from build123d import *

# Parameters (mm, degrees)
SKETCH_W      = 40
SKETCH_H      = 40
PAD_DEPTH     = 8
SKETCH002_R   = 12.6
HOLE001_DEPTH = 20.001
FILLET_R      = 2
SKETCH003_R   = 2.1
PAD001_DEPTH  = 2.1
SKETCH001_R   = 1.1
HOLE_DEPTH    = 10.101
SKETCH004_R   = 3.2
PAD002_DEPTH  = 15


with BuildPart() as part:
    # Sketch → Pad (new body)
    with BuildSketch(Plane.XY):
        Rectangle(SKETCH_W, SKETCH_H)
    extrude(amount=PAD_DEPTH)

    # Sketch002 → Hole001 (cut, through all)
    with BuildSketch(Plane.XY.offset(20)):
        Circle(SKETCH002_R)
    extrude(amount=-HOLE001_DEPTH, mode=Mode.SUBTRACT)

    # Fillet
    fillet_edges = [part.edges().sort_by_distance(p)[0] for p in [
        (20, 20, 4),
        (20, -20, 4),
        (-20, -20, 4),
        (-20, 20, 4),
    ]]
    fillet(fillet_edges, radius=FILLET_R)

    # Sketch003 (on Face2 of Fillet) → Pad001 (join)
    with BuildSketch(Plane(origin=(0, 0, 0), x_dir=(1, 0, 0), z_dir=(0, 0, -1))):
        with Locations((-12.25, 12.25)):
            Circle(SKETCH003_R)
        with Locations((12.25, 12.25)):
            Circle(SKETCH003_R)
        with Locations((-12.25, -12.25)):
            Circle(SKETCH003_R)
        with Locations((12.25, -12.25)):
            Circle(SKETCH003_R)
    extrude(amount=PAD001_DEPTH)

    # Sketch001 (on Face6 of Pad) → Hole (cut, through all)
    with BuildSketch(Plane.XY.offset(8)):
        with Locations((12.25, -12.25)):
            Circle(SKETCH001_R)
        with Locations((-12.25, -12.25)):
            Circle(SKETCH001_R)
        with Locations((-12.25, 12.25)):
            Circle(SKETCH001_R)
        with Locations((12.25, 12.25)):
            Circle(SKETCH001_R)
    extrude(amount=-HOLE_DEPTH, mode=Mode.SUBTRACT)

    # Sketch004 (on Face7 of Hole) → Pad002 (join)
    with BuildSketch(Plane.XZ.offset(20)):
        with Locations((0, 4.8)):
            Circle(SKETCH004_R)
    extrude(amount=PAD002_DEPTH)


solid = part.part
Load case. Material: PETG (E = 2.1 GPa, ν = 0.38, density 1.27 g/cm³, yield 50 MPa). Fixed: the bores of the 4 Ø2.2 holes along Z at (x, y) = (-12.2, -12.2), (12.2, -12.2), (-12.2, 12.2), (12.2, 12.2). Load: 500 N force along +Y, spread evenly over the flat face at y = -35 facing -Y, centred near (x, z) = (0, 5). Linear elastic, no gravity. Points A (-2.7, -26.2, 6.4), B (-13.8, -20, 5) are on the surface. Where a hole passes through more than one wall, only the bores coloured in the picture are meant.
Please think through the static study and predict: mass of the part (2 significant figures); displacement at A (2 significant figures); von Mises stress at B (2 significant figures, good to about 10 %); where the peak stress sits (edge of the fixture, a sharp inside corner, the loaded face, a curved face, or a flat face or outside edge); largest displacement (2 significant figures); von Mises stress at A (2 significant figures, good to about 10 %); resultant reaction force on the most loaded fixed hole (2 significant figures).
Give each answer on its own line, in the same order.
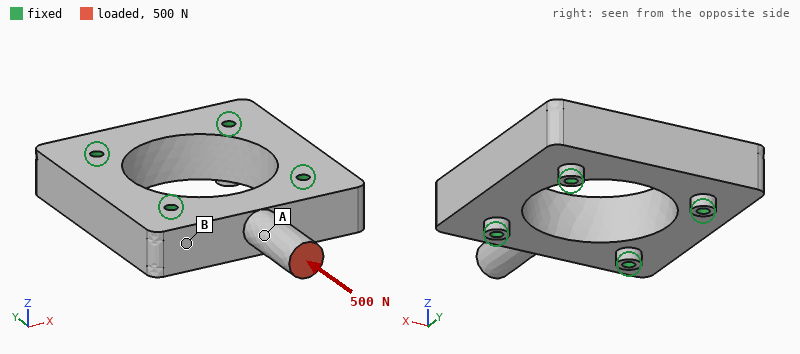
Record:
12 g
0.16 mm
2.4 MPa
a flat face or outside edge
0.24 mm
15 MPa
340 N
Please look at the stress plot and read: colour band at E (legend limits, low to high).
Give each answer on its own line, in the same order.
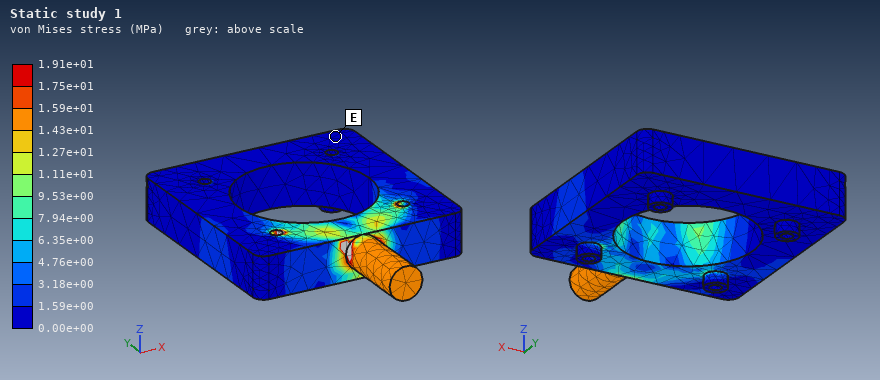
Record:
0.00e+00 to 1.59e+00 MPa
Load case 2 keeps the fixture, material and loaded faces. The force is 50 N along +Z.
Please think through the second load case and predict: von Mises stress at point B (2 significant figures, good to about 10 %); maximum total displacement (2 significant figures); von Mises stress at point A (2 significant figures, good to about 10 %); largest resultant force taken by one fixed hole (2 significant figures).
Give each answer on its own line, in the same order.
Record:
1.5 MPa
0.70 mm
9.3 MPa
29 N
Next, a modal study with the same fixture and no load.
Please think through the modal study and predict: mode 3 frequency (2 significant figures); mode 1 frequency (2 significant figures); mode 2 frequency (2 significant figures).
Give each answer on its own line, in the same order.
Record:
8900 Hz
3000 Hz
3900 Hz
